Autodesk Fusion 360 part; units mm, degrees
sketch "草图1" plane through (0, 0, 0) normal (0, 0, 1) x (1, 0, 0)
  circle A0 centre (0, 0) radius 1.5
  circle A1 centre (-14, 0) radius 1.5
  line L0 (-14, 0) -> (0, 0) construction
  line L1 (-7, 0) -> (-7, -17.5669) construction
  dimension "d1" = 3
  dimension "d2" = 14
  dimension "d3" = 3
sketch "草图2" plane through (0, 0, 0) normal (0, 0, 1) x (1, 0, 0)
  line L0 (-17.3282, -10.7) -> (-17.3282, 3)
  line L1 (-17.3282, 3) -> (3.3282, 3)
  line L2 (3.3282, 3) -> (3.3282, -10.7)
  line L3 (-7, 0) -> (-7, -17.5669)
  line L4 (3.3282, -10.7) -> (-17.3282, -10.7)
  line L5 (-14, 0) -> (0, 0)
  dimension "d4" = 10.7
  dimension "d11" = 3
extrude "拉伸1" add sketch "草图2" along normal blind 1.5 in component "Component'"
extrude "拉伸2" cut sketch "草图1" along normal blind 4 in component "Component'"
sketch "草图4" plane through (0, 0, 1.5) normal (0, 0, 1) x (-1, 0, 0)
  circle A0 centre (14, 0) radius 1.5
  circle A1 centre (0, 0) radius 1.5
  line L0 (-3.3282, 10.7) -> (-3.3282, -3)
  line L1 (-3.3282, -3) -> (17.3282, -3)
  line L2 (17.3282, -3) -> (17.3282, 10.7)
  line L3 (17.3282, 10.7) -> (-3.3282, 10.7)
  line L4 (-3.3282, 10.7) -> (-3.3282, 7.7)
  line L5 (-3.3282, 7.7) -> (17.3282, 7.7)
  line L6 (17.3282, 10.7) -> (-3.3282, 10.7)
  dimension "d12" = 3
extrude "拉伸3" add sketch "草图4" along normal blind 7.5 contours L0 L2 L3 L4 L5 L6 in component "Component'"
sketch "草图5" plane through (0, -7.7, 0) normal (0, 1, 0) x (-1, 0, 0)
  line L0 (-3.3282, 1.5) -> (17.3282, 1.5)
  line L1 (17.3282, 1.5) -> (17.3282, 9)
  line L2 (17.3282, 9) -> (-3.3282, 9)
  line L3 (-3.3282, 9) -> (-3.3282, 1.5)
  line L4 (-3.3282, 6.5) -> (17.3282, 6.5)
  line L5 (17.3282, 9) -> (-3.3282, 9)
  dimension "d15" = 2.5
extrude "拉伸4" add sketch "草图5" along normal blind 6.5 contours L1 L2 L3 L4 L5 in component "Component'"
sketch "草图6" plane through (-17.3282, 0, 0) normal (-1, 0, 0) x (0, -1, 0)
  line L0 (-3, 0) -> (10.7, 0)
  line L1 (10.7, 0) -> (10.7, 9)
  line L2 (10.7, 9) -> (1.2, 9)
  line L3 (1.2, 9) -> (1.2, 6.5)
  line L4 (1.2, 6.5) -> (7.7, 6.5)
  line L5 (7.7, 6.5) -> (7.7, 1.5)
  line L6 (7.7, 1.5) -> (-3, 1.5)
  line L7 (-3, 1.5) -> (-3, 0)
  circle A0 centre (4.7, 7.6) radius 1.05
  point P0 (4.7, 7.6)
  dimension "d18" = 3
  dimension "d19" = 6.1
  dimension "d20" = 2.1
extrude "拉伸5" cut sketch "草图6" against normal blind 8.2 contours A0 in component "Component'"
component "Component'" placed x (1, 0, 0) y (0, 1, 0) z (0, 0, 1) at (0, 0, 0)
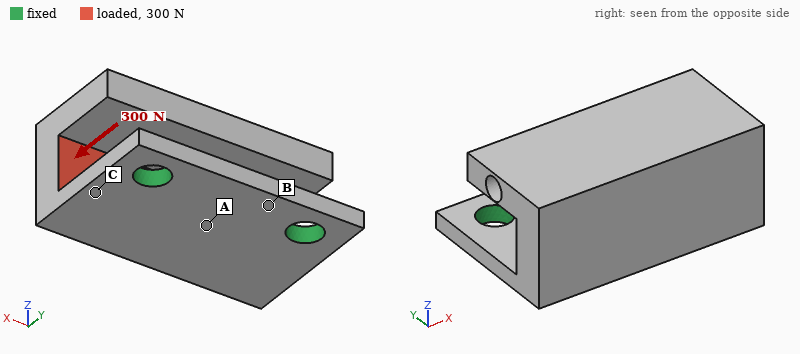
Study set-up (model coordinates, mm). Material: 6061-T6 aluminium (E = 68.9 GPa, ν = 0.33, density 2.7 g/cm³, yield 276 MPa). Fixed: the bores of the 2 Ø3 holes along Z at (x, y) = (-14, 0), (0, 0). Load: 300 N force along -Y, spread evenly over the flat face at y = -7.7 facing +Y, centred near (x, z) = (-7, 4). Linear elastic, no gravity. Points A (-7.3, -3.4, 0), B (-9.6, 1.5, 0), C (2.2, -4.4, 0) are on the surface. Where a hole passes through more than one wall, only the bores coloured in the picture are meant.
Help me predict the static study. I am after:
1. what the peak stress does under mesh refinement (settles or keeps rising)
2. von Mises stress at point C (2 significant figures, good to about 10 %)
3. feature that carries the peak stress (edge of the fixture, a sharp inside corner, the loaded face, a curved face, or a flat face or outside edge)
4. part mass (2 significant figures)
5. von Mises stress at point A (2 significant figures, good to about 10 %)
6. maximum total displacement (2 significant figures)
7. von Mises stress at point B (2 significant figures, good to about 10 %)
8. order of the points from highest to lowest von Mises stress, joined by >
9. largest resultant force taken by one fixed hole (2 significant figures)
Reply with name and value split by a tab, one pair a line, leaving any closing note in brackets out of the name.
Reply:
what the peak stress does under mesh refinement	keeps rising
von Mises stress at point C	120 MPa
feature that carries the peak stress	edge of the fixture
part mass	3.2 g
von Mises stress at point A	85 MPa
maximum total displacement	0.19 mm
von Mises stress at point B	22 MPa
order of the points from highest to lowest von Mises stress, joined by >	C > A > B
largest resultant force taken by one fixed hole	150 N
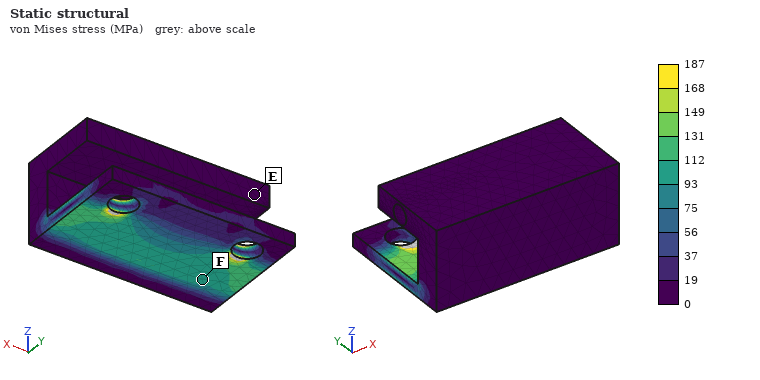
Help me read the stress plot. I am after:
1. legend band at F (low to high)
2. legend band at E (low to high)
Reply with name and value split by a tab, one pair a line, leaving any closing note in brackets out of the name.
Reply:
legend band at F	93 to 112 MPa
legend band at E	0 to 19 MPa
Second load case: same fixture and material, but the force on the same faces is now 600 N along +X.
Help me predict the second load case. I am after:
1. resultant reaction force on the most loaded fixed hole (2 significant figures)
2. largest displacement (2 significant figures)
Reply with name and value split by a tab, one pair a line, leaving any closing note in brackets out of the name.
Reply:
resultant reaction force on the most loaded fixed hole	430 N
largest displacement	82 µm
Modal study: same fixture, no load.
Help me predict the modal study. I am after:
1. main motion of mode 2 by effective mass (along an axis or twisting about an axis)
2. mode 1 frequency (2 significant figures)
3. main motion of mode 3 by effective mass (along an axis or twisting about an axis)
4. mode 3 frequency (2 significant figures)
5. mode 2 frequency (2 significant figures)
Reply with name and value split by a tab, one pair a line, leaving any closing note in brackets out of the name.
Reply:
main motion of mode 2 by effective mass	along X
mode 1 frequency	3400 Hz
main motion of mode 3 by effective mass	along Z
mode 3 frequency	9800 Hz
mode 2 frequency	7200 Hz
